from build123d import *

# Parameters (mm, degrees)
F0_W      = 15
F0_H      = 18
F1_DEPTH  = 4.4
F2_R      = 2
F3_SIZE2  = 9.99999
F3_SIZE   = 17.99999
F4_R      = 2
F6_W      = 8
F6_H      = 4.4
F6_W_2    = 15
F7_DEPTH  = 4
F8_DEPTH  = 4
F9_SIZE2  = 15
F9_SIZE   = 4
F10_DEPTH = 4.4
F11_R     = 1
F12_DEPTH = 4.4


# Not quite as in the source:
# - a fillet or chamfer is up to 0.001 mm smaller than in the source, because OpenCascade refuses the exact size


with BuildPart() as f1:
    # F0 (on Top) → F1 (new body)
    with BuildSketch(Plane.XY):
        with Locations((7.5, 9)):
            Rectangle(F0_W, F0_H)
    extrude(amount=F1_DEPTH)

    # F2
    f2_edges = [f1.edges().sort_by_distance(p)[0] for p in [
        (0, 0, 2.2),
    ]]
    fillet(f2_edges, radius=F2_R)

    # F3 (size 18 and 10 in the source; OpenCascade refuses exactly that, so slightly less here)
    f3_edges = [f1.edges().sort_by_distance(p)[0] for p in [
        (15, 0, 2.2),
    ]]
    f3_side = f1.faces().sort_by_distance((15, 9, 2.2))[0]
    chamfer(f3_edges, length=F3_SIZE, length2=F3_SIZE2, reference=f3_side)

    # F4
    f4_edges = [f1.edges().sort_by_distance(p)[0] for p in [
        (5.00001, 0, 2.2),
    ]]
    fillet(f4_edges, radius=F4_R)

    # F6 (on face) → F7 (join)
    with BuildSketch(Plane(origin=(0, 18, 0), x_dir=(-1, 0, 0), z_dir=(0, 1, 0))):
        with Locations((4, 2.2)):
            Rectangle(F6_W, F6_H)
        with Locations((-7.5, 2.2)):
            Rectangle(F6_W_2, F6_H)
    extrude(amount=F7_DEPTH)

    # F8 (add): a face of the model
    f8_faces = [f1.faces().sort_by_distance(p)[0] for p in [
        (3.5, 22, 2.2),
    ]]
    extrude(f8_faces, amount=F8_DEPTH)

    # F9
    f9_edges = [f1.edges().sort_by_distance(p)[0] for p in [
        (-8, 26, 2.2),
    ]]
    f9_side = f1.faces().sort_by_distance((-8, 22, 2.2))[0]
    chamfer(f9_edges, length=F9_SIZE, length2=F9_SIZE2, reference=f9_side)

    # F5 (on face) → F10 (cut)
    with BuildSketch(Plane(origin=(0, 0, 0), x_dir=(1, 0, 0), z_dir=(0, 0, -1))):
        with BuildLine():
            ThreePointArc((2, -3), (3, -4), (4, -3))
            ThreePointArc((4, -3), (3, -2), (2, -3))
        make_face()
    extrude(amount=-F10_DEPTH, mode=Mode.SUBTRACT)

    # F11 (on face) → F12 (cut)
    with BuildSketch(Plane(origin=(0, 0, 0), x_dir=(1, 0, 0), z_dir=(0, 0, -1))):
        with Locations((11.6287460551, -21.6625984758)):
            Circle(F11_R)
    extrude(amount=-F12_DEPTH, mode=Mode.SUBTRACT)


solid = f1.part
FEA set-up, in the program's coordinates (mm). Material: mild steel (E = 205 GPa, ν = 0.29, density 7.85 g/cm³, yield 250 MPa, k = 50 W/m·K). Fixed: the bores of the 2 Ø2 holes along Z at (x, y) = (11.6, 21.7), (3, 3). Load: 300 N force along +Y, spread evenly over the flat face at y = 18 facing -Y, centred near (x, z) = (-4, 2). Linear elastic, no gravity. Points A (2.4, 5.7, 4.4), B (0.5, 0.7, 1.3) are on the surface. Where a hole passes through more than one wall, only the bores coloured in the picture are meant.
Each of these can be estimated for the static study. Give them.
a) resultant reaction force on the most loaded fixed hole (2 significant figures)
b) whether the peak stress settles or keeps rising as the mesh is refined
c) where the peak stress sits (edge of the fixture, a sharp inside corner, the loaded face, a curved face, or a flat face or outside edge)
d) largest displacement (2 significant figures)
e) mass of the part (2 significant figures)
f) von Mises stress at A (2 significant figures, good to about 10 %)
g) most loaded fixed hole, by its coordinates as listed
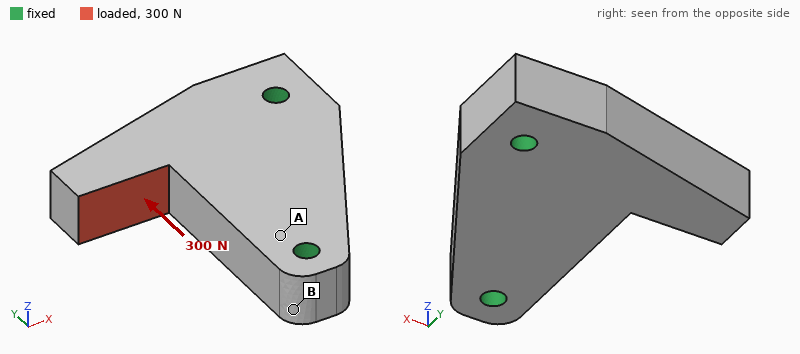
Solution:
290 N
keeps rising
a sharp inside corner
6.8 µm
11 g
18 MPa
(3, 3)
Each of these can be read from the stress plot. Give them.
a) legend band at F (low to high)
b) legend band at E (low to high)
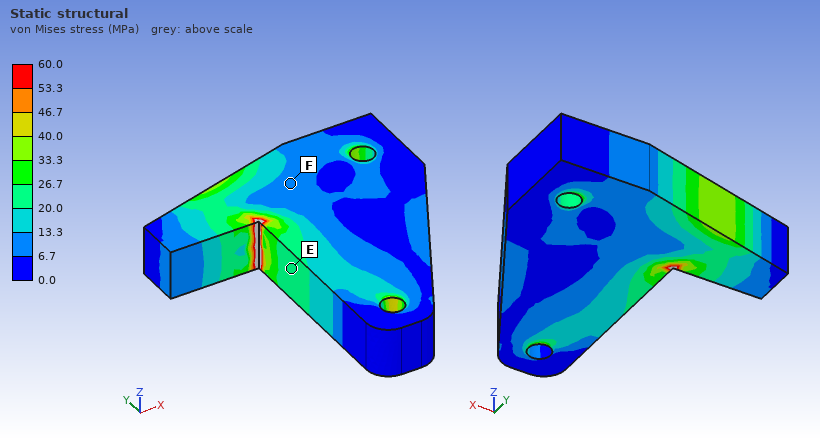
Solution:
6.7 to 13.3 MPa
20.0 to 26.7 MPa
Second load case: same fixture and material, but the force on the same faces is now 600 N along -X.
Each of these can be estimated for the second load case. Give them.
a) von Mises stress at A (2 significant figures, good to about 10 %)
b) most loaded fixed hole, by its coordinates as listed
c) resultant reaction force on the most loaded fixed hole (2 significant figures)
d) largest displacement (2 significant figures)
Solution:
7.7 MPa
(11.6, 21.7)
510 N
7.4 µm
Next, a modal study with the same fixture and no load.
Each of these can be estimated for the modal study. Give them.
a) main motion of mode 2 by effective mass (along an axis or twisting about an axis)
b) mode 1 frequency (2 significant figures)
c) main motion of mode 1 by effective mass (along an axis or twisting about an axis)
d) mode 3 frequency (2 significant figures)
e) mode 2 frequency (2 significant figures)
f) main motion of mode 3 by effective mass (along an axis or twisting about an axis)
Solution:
along Y
14 kHz
along Z
40 kHz
32 kHz
along Z
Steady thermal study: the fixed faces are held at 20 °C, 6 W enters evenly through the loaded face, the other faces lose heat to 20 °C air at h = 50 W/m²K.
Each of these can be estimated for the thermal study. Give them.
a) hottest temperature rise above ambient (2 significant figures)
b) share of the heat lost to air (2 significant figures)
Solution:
52 K
9.2 %
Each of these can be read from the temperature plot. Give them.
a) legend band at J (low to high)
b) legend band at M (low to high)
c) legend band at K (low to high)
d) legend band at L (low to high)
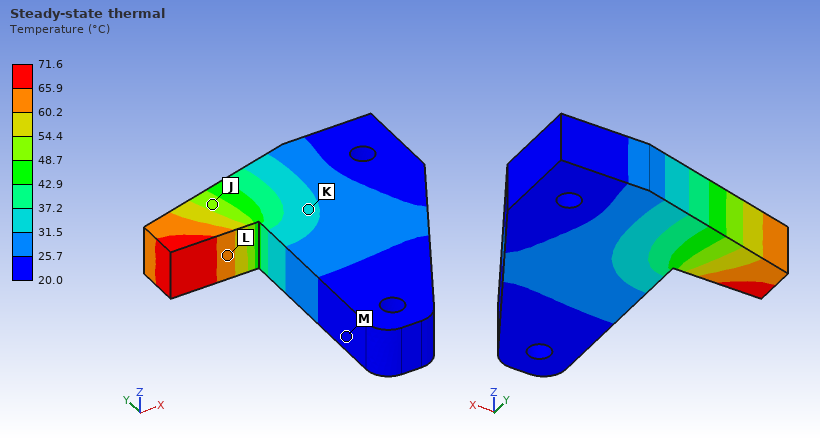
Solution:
48.7 to 54.4 °C
20.0 to 25.7 °C
31.5 to 37.2 °C
60.2 to 65.9 °C
